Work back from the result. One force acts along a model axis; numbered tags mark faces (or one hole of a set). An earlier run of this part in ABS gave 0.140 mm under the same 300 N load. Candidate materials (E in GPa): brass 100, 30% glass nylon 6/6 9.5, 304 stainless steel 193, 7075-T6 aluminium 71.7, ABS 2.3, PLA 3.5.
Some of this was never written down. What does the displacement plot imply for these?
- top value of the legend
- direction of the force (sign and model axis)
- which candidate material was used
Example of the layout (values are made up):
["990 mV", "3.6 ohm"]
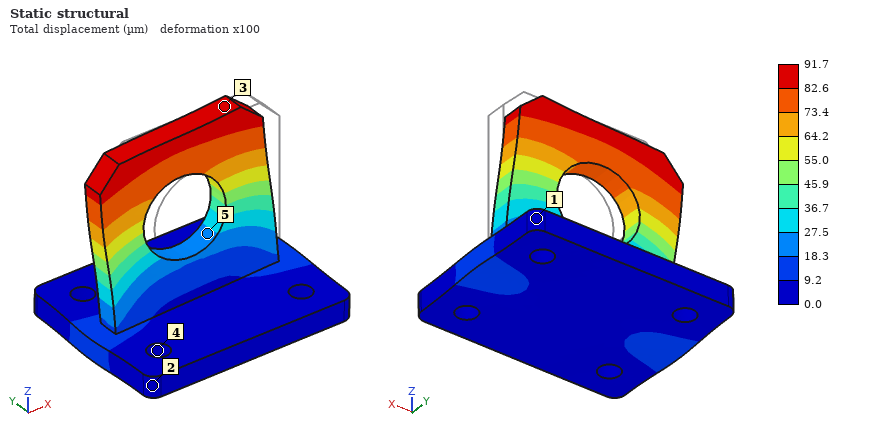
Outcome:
["91.7 µm", "-X", "PLA"]
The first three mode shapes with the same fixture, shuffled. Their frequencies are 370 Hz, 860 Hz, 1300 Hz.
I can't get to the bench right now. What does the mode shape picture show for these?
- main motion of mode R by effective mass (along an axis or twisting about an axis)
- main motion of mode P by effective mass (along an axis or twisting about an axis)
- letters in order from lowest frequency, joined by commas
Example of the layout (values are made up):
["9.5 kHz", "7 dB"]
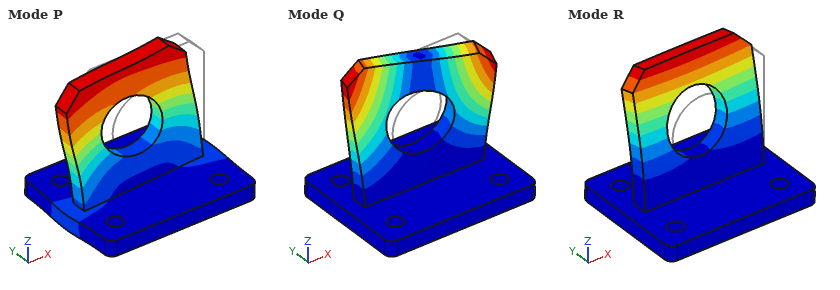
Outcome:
["along Y", "along X", "R, Q, P"]
